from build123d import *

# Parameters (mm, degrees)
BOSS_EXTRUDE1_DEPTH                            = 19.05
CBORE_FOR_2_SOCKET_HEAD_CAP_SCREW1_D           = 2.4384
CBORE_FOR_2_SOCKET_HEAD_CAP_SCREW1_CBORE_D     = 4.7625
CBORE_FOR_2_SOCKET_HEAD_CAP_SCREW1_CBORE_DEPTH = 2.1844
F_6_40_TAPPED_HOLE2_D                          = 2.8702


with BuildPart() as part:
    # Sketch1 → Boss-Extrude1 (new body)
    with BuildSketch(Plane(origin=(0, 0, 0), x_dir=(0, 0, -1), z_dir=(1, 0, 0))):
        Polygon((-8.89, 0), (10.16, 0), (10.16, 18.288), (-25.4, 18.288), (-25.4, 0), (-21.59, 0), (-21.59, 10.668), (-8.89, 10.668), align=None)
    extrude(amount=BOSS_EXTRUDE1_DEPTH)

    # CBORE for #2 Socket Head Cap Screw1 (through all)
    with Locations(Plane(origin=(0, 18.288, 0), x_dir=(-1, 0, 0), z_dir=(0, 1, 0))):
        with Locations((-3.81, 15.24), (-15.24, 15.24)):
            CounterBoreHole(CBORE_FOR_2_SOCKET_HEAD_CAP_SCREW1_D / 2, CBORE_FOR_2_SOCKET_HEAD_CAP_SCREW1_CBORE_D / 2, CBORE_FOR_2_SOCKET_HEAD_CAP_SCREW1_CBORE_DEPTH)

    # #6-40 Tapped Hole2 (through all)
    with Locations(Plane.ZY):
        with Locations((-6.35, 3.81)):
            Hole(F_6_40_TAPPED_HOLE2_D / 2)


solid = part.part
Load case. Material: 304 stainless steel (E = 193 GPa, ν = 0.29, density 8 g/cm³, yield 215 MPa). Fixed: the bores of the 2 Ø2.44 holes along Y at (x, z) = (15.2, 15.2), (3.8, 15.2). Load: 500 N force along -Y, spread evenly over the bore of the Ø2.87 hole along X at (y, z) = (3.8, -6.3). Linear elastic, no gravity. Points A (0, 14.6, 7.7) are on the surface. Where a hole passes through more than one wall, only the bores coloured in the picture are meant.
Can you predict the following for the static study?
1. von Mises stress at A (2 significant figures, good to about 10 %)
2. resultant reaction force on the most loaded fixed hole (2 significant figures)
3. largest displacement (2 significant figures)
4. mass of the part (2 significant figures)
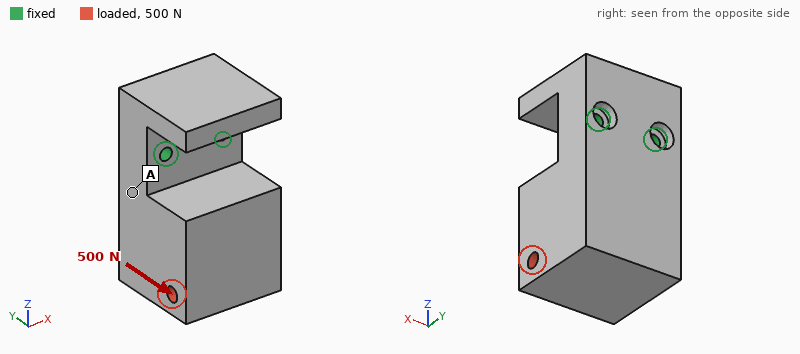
21 MPa
260 N
26 µm
76 g
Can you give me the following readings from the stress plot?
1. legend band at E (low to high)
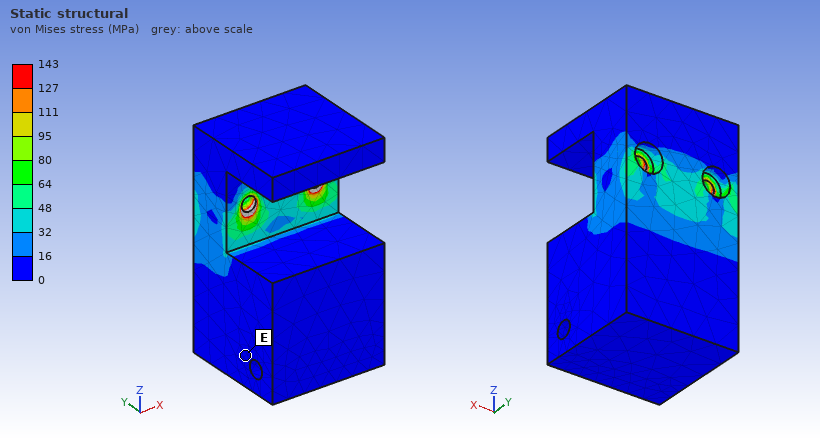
0 to 16 MPa
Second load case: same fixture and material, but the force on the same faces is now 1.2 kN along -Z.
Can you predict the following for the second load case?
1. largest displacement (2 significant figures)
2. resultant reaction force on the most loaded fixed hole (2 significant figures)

34 µm
610 N
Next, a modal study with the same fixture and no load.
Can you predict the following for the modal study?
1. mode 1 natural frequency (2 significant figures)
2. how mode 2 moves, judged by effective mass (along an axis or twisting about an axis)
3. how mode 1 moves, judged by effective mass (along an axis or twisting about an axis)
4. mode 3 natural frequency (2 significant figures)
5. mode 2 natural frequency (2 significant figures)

4300 Hz
along X
along Y
14 kHz
9300 Hz
